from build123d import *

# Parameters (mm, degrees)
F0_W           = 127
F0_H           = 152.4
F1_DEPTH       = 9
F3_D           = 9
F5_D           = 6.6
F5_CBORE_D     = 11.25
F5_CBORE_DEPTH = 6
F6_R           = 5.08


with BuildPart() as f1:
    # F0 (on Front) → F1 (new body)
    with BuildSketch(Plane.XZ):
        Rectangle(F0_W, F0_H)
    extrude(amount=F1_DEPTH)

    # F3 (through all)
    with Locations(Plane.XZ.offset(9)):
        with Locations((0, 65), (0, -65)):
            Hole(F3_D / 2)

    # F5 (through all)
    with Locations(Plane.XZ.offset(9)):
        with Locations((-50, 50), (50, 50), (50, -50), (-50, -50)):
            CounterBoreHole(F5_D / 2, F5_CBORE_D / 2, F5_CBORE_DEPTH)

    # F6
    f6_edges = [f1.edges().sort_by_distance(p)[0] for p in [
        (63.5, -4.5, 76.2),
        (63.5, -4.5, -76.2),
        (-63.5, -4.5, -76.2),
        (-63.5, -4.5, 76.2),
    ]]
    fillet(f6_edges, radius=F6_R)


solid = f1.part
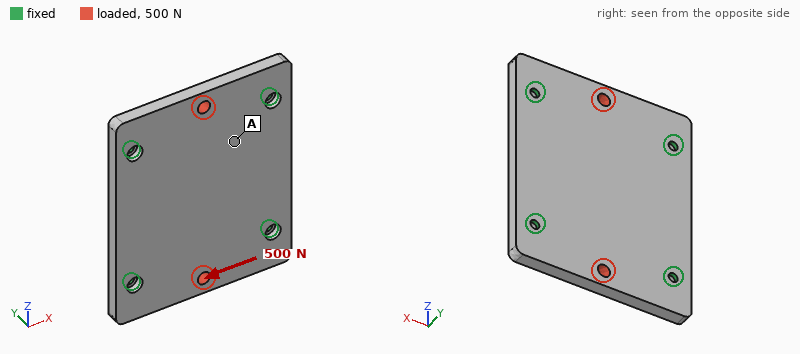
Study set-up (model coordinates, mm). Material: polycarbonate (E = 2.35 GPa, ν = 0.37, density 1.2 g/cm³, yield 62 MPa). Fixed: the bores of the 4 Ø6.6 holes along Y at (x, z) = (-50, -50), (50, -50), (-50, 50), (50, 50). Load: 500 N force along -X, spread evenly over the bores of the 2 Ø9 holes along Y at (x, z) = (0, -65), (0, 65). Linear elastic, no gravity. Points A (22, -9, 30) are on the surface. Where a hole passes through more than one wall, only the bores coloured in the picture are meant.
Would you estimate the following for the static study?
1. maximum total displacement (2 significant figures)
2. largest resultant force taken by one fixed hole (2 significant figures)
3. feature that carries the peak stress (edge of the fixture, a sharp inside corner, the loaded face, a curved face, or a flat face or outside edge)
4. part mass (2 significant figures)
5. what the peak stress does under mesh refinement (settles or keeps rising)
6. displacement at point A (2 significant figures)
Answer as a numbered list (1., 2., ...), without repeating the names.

1. 21 µm
2. 130 N
3. edge of the fixture
4. 200 g
5. keeps rising
6. 8.0 µm
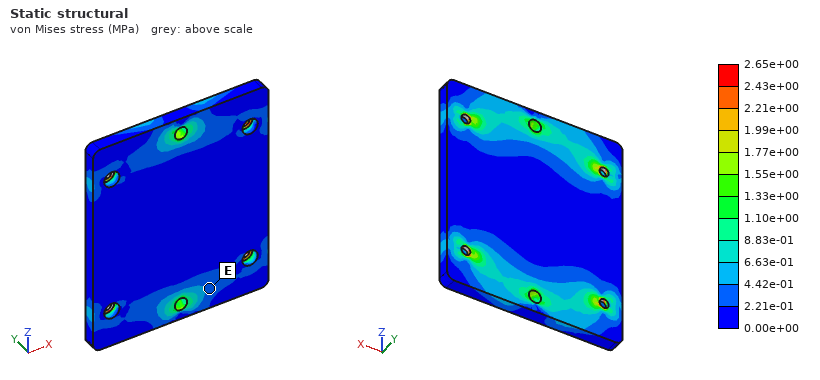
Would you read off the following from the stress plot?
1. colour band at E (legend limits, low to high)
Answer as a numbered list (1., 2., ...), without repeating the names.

1. 2.21e-01 to 4.42e-01 MPa
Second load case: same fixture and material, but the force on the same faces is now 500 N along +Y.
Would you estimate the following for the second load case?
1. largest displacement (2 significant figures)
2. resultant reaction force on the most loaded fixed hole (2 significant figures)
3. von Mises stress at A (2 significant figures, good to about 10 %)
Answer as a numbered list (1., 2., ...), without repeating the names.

1. 0.67 mm
2. 330 N
3. 2.9 MPa
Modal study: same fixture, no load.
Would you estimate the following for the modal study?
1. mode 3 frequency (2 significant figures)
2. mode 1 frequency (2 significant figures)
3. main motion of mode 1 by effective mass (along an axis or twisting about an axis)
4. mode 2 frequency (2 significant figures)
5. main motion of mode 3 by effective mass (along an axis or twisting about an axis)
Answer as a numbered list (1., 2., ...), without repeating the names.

1. 880 Hz
2. 680 Hz
3. along Y
4. 850 Hz
5. twisting about X
